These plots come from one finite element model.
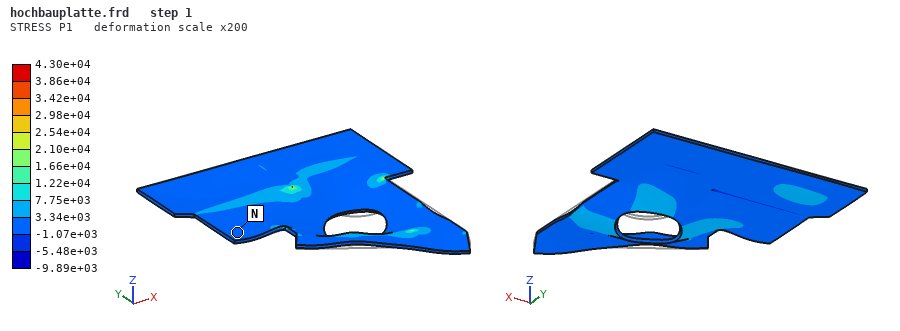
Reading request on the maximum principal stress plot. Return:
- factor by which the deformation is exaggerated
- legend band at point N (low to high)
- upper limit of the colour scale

200
-1.07e+03 to 3.34e+03
4.30e+04
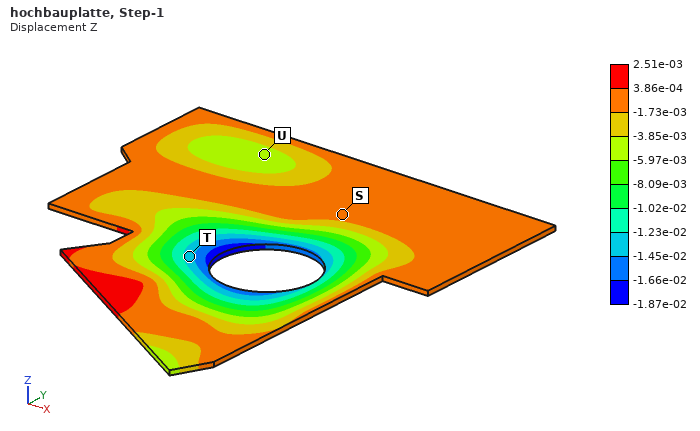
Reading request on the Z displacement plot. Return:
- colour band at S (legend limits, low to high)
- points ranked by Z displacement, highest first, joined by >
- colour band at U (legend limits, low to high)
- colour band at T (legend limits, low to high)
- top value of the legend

-1.73e-03 to 3.86e-04
S > U > T
-5.97e-03 to -3.85e-03
-1.45e-02 to -1.23e-02
2.51e-03
